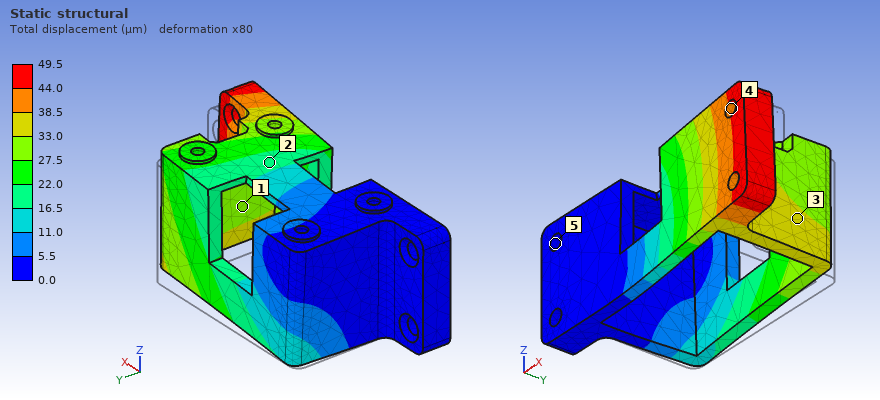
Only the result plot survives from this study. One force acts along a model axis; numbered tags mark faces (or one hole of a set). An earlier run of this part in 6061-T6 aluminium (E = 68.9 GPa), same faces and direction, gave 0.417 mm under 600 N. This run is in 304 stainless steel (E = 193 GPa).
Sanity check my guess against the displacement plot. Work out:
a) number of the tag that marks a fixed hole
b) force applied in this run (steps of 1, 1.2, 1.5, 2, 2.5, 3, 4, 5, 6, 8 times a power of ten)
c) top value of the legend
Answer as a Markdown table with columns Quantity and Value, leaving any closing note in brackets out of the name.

| Quantity | Value |
|---|---|
| number of the tag that marks a fixed hole | 5 |
| force applied in this run | 200 N |
| top value of the legend | 49.5 µm |
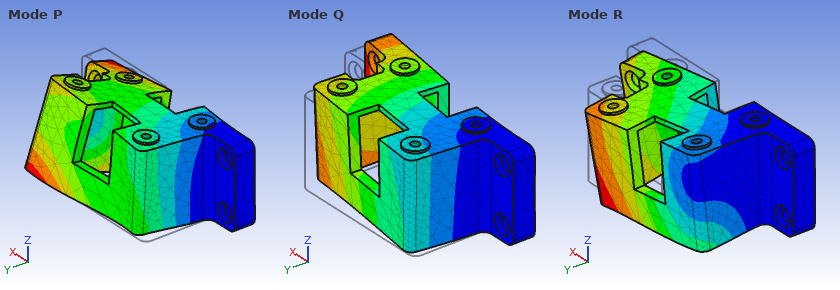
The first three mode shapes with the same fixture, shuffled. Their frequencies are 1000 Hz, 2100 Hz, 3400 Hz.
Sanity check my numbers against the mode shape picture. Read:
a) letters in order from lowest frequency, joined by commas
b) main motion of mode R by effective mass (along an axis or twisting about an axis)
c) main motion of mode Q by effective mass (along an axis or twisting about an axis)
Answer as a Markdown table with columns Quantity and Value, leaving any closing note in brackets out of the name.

| Quantity | Value |
|---|---|
| letters in order from lowest frequency, joined by commas | Q, R, P |
| main motion of mode R by effective mass | along Z |
| main motion of mode Q by effective mass | along Y |
